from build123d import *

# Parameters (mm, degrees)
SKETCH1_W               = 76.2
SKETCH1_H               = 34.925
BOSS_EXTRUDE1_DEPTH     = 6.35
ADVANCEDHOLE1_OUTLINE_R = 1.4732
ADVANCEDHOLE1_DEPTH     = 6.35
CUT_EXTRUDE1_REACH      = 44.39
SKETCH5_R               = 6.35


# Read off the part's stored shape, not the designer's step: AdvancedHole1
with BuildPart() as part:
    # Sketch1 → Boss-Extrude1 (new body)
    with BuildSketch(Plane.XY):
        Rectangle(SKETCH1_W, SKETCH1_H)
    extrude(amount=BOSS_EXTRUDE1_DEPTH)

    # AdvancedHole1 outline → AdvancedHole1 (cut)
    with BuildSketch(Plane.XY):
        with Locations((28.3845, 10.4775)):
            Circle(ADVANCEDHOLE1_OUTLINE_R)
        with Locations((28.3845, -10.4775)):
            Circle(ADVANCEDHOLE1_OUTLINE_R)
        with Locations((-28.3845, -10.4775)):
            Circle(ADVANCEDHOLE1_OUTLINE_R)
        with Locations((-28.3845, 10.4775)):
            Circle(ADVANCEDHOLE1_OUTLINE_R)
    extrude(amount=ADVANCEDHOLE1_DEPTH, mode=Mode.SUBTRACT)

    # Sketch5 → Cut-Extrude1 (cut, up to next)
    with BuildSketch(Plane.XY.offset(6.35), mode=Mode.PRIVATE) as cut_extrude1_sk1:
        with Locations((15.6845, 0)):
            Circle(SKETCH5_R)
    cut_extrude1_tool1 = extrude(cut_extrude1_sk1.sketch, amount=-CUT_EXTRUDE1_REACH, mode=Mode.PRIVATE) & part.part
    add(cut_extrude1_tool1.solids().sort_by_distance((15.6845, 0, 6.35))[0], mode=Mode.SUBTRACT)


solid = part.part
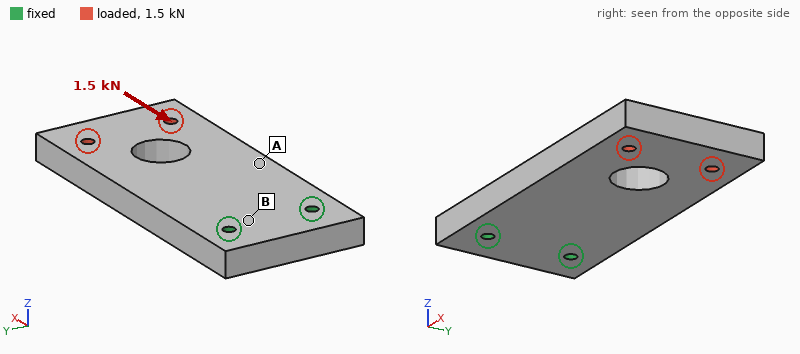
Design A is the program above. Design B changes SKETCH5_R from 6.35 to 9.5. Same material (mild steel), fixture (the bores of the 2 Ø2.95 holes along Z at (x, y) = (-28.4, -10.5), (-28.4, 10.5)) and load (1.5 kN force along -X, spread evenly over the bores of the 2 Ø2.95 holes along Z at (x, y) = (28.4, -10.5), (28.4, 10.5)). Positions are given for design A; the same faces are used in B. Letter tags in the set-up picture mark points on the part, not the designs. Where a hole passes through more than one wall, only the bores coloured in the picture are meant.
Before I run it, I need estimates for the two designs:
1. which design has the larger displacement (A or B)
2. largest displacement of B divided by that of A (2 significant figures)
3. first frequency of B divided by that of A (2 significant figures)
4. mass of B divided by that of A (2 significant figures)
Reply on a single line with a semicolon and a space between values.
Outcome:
B; 1.3; 1.0; 0.94
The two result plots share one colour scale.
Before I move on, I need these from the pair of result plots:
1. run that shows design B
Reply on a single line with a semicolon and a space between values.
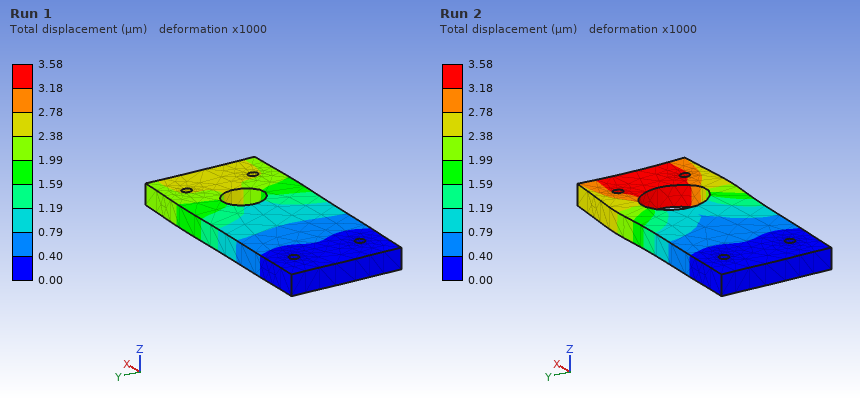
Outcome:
Run 2
